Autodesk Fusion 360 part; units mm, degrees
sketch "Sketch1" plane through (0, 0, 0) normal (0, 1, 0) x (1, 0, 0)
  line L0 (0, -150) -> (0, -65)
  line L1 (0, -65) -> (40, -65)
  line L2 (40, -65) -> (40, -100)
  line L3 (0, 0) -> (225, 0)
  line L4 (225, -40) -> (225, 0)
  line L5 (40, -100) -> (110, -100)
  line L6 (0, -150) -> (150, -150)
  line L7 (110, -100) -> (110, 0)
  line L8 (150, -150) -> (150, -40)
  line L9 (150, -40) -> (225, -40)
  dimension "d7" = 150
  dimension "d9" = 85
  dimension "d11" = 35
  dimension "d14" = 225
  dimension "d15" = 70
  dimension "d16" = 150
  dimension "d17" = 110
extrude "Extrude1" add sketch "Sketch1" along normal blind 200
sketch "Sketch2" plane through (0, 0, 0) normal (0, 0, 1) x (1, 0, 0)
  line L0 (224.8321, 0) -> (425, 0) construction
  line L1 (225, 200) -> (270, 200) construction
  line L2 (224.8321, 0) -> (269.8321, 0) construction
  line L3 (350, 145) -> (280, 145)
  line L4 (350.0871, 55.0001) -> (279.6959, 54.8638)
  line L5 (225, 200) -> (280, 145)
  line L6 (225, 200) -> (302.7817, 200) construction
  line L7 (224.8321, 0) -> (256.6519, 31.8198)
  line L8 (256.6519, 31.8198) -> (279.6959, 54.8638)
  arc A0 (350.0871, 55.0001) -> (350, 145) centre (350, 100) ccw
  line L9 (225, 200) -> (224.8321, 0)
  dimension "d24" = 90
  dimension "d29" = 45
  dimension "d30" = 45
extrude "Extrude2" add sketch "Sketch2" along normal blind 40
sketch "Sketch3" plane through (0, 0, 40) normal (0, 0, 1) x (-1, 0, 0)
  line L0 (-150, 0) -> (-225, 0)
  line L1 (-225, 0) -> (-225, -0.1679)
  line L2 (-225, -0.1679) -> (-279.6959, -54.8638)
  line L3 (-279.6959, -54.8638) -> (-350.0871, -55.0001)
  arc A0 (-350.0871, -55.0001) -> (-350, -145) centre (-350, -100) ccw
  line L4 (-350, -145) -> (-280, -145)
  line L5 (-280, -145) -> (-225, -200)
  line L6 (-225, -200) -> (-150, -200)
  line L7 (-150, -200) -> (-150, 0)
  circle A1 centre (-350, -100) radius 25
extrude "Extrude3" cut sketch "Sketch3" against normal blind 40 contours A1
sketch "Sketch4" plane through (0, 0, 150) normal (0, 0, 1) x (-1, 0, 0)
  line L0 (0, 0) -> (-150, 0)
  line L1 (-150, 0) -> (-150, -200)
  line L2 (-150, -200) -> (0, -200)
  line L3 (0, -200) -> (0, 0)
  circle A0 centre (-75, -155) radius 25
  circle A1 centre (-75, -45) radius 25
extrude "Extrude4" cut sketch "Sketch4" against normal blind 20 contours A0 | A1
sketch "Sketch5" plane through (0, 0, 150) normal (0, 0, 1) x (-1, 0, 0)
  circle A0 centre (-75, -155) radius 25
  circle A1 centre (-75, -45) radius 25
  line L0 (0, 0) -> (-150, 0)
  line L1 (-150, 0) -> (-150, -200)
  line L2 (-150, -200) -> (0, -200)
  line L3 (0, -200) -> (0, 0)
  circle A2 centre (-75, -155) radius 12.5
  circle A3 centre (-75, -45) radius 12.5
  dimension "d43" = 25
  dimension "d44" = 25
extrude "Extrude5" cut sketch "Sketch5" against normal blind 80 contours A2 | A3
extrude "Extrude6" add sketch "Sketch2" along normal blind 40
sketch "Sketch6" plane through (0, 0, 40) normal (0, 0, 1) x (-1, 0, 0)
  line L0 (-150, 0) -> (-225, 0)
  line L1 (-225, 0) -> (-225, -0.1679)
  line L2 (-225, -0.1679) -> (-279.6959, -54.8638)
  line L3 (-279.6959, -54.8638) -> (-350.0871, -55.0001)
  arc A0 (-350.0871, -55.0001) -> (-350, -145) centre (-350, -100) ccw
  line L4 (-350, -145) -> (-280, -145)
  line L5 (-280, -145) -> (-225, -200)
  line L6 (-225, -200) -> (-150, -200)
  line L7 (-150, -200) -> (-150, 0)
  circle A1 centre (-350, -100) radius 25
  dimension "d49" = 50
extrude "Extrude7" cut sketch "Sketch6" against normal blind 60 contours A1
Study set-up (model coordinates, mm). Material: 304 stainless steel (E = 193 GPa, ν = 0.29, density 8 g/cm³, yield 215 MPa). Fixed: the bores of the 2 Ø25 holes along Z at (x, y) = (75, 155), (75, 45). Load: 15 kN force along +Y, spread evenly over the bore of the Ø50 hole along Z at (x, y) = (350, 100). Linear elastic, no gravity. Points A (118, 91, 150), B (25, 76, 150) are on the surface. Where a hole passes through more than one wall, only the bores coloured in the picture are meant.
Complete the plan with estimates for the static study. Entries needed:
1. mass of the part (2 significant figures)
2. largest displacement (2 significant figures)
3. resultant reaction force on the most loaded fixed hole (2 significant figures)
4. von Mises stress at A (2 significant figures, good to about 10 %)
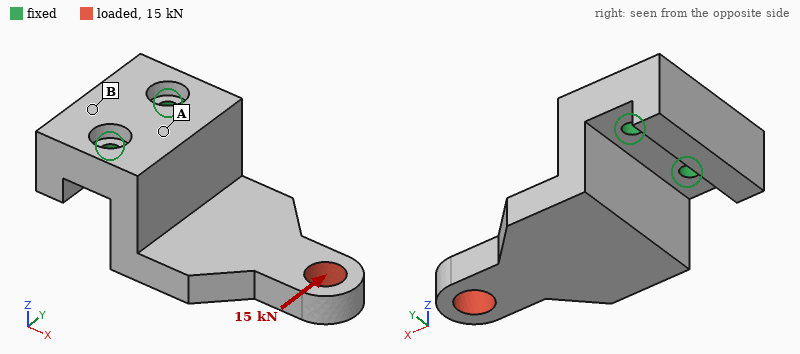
30 kg
0.20 mm
37 kN
12 MPa
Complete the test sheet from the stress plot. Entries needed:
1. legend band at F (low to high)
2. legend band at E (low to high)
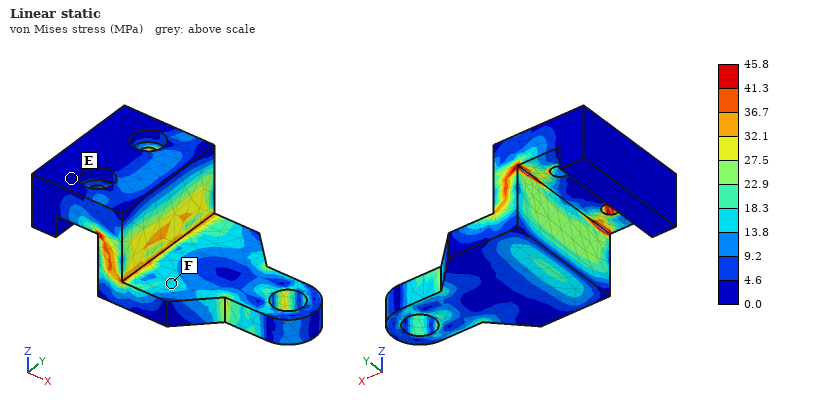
13.8 to 18.3 MPa
0.0 to 4.6 MPa
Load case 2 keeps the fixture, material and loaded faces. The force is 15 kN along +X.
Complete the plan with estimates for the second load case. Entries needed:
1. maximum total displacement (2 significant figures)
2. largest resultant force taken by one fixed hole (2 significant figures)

0.21 mm
7.7 kN
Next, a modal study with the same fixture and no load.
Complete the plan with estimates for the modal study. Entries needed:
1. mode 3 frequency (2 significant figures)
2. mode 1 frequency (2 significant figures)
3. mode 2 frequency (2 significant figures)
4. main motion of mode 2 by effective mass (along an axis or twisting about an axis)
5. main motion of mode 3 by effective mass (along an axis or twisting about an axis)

1200 Hz
350 Hz
840 Hz
along Y
along X
